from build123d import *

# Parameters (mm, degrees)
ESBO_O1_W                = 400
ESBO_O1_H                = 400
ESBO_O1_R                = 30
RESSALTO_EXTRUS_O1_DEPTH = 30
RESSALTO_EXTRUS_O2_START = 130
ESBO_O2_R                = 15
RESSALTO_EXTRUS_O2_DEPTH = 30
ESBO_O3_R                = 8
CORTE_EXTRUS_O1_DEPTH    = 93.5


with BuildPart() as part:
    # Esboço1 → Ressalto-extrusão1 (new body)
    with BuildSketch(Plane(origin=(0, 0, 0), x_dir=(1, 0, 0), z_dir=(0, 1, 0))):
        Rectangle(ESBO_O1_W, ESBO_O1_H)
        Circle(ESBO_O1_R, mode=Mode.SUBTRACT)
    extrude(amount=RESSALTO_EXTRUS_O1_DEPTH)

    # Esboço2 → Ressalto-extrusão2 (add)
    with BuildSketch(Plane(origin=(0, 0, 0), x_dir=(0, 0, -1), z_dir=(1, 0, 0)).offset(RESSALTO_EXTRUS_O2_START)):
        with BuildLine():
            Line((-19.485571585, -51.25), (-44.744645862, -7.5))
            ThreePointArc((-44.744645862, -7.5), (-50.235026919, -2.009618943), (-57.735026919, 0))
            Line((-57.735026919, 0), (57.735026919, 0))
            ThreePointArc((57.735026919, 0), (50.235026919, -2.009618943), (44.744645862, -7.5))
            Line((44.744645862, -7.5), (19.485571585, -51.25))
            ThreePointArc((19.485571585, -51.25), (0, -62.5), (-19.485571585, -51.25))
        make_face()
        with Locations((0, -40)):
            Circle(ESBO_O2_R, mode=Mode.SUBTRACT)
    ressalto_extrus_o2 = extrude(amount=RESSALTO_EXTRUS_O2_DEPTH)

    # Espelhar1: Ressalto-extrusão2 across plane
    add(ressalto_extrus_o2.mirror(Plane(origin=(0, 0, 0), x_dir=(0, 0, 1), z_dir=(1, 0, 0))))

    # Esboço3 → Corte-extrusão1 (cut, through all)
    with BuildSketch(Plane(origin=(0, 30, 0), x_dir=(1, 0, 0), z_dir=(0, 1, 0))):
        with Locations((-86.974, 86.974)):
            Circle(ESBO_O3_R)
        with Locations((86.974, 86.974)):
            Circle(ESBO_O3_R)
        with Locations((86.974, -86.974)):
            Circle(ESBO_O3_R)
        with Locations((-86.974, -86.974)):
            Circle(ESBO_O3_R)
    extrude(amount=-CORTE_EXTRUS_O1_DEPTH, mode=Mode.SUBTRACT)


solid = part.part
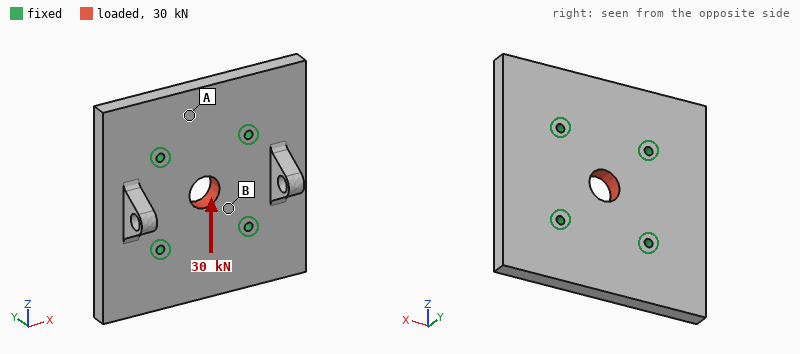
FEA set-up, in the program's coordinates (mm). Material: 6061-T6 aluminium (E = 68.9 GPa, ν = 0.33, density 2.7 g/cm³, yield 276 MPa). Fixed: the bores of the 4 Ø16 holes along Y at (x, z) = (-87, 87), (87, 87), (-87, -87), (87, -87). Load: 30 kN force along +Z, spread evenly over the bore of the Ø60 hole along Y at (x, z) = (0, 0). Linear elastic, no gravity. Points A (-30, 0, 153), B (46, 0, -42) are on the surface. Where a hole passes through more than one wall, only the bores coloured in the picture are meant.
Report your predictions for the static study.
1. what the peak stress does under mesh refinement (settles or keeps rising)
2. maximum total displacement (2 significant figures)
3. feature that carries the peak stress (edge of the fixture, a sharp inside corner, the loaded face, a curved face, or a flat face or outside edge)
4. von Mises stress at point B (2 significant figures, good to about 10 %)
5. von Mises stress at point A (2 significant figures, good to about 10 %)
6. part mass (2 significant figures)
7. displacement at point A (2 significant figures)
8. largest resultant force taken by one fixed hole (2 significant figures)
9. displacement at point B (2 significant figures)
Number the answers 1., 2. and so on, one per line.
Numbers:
1. keeps rising
2. 7.5 µm
3. edge of the fixture
4. 3.8 MPa
5. 1.2 MPa
6. 13 kg
7. 2.9 µm
8. 7.8 kN
9. 3.9 µm
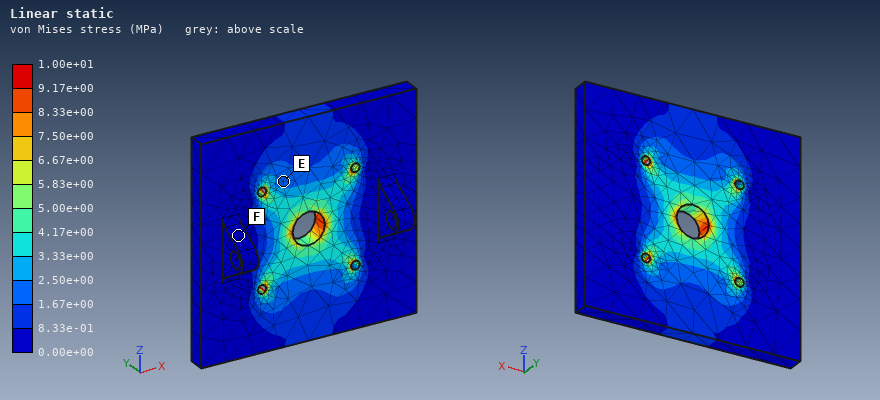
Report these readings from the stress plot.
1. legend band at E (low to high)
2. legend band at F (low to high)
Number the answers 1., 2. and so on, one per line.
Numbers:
1. 1.67e+00 to 2.50e+00 MPa
2. 0.00e+00 to 8.33e-01 MPa
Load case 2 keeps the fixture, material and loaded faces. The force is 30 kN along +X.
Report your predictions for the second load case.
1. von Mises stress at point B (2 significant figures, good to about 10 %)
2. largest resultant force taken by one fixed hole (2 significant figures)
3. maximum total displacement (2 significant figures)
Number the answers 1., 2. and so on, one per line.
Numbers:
1. 3.9 MPa
2. 7.8 kN
3. 7.5 µm
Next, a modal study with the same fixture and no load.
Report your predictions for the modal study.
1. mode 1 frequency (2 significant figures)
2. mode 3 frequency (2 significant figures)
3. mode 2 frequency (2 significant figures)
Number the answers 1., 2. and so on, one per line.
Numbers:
1. 1300 Hz
2. 1400 Hz
3. 1300 Hz
